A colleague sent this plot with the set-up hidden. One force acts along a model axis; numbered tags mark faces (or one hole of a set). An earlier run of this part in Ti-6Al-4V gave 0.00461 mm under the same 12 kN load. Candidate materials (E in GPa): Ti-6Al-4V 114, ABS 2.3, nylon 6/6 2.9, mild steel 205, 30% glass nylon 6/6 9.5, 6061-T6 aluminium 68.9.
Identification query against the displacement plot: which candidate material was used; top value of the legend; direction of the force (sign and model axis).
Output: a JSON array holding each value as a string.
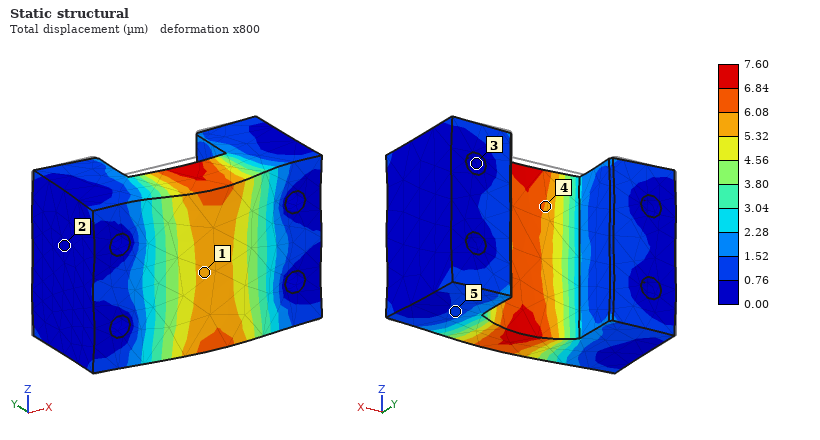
["6061-T6 aluminium", "7.60 µm", "-Y"]
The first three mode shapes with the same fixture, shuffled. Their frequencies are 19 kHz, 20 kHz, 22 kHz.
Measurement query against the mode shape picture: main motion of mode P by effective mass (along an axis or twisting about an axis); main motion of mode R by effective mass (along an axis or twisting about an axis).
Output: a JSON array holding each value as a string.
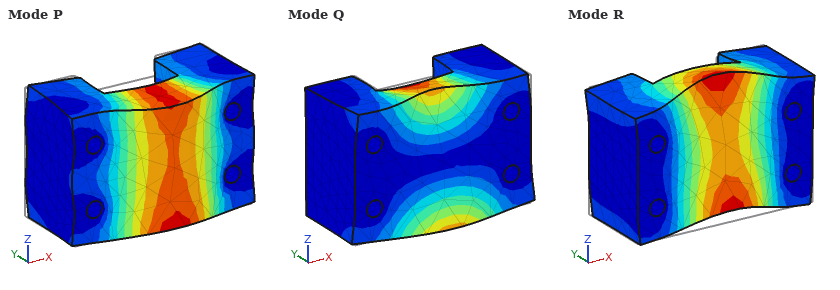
["along Y", "along Z"]
